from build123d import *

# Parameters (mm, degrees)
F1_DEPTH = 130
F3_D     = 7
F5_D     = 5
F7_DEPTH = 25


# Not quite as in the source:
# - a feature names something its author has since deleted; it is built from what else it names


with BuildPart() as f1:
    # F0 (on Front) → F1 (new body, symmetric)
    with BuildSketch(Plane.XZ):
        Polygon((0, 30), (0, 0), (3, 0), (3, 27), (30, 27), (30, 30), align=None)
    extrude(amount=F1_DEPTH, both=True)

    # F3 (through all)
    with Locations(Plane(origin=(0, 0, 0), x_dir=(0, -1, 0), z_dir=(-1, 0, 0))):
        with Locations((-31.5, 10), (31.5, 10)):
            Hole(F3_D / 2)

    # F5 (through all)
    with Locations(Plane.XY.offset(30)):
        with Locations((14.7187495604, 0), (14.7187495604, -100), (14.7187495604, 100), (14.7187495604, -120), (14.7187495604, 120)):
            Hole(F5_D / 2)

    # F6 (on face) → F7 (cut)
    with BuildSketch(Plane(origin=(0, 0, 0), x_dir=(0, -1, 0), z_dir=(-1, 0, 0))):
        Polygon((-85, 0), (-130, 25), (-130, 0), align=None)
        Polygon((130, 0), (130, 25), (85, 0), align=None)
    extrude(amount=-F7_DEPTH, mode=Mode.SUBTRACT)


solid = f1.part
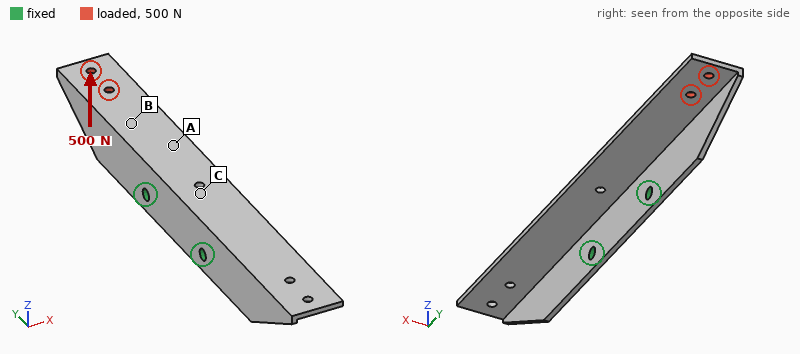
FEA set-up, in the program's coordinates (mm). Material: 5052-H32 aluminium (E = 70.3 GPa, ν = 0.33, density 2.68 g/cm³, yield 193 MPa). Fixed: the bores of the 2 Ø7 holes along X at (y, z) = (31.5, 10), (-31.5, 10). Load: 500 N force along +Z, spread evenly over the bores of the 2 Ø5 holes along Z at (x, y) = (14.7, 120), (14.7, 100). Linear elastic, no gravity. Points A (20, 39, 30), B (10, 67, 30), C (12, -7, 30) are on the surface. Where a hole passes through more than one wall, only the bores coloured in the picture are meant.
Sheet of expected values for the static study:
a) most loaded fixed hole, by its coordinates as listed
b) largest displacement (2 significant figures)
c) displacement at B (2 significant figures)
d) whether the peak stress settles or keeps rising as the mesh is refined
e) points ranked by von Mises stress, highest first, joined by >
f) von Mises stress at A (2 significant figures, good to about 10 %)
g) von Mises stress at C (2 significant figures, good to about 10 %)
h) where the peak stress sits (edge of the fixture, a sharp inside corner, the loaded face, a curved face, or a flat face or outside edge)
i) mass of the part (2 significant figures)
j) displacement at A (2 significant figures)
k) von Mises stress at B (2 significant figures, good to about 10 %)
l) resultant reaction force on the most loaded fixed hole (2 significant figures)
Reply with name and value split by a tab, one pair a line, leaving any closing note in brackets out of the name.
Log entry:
most loaded fixed hole, by its coordinates as listed	(31.5, 10)
largest displacement	1.7 mm
displacement at B	0.34 mm
whether the peak stress settles or keeps rising as the mesh is refined	keeps rising
points ranked by von Mises stress, highest first, joined by >	B > A > C
von Mises stress at A	44 MPa
von Mises stress at C	15 MPa
where the peak stress sits	edge of the fixture
mass of the part	110 g
displacement at A	0.26 mm
von Mises stress at B	62 MPa
resultant reaction force on the most loaded fixed hole	1.2 kN
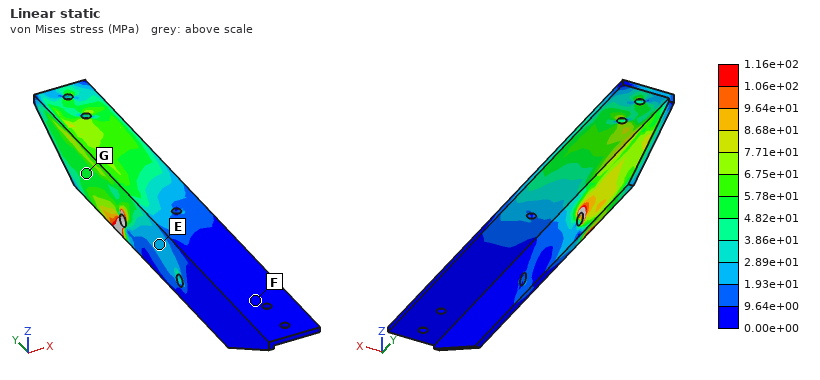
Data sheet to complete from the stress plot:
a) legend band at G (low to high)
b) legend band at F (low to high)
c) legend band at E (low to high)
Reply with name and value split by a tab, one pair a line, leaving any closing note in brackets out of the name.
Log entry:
legend band at G	4.82e+01 to 5.78e+01 MPa
legend band at F	0.00e+00 to 9.64e+00 MPa
legend band at E	1.93e+01 to 2.89e+01 MPa
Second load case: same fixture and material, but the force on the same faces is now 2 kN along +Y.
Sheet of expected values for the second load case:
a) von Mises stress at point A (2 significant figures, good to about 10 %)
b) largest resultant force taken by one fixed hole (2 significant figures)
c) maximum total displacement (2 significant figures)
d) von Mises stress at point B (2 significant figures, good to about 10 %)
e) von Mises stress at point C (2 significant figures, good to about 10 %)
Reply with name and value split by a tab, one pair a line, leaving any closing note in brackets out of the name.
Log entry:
von Mises stress at point A	31 MPa
largest resultant force taken by one fixed hole	1.2 kN
maximum total displacement	0.40 mm
von Mises stress at point B	19 MPa
von Mises stress at point C	12 MPa
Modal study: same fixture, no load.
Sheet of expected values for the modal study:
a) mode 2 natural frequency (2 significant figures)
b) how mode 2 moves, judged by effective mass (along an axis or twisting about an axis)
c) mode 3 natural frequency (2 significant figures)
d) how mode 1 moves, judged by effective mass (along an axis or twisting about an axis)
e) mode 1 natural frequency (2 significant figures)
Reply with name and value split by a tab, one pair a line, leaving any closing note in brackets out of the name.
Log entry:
mode 2 natural frequency	860 Hz
how mode 2 moves, judged by effective mass	along Z
mode 3 natural frequency	1100 Hz
how mode 1 moves, judged by effective mass	twisting about Z
mode 1 natural frequency	680 Hz
